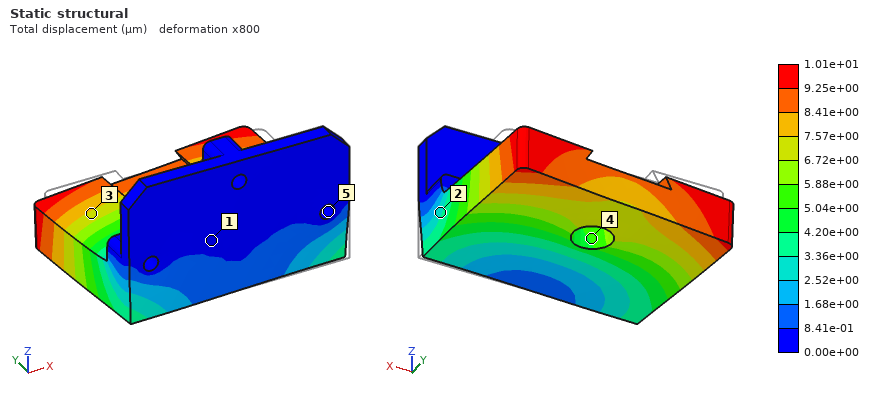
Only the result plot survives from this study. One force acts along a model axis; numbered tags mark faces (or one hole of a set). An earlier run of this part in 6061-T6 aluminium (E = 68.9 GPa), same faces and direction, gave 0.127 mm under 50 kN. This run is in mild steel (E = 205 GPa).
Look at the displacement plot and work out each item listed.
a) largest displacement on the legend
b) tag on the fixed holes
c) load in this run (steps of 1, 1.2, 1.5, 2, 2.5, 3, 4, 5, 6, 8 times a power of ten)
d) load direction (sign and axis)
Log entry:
1.01e+01 µm
5
12 kN
-X
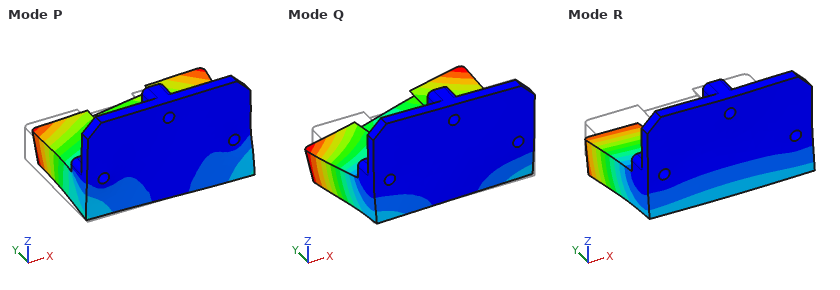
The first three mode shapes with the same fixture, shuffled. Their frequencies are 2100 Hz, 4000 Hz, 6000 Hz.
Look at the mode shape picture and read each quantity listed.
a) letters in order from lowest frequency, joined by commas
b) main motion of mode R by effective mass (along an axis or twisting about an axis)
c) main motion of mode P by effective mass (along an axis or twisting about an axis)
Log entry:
R, Q, P
along Z
along X
